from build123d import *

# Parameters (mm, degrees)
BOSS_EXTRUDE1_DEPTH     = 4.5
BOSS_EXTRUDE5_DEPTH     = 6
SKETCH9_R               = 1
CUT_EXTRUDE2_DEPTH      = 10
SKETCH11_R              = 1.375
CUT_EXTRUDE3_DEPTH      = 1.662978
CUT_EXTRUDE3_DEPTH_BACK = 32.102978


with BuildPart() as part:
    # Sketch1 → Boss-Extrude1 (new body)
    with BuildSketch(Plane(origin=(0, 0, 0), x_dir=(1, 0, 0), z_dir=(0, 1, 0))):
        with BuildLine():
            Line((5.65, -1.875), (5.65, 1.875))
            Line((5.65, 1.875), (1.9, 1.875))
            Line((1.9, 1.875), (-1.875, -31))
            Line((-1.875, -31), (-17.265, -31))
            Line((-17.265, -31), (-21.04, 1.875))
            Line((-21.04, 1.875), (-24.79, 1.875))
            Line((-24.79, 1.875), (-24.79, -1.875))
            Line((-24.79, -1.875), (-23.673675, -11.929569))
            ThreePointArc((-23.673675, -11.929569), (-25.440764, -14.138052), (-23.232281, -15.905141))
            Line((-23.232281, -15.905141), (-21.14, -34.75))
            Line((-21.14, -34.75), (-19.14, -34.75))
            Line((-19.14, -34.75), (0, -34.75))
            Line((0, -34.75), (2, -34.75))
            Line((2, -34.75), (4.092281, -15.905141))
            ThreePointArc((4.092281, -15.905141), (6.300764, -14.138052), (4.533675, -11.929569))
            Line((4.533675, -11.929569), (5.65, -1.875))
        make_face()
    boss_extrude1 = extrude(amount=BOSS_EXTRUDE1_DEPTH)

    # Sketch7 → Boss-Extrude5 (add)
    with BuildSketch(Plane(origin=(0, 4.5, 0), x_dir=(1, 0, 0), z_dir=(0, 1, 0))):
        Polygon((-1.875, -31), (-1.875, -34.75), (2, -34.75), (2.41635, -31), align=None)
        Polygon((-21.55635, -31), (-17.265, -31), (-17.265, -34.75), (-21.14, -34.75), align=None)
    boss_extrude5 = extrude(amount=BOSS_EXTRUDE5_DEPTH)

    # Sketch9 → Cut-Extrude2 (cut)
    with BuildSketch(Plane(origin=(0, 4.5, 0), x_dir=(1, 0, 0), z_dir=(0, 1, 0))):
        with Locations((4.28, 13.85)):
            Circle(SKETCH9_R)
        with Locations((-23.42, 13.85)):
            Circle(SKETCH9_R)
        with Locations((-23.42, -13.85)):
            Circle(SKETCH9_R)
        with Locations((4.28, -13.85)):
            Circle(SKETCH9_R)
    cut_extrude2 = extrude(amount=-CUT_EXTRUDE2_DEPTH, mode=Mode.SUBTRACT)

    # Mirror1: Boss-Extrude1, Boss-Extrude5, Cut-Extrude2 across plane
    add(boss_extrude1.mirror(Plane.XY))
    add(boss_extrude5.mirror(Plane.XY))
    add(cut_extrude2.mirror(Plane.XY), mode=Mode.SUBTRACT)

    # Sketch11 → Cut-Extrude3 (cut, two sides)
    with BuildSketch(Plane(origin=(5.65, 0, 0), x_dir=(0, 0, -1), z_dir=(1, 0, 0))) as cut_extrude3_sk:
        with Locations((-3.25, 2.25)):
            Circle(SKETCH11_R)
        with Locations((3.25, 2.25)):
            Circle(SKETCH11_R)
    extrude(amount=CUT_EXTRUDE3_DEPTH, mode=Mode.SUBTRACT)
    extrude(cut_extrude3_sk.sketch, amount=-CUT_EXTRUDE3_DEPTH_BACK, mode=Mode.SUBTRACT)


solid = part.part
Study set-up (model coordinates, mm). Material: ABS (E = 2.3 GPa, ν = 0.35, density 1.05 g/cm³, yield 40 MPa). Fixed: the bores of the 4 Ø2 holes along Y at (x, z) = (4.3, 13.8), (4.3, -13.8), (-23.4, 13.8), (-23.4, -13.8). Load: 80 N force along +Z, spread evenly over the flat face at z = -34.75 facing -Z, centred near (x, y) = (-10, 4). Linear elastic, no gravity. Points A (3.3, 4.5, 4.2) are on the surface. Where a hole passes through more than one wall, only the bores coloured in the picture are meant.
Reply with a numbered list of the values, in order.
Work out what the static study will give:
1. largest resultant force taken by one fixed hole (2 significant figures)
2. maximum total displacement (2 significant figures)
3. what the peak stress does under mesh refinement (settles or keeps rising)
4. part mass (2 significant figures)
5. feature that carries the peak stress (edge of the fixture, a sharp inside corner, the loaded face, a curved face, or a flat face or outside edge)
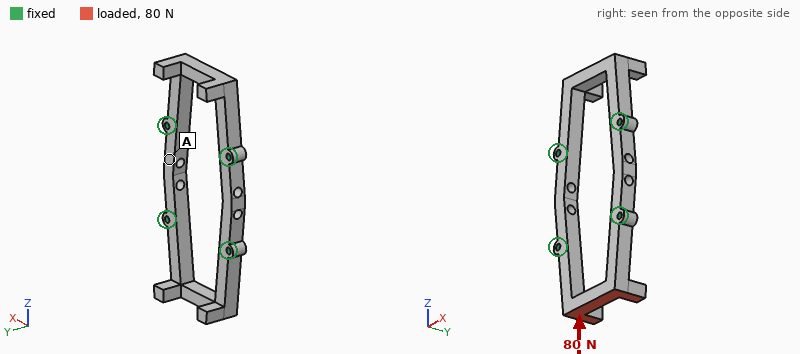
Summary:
1. 40 N
2. 0.27 mm
3. keeps rising
4. 3.7 g
5. edge of the fixture
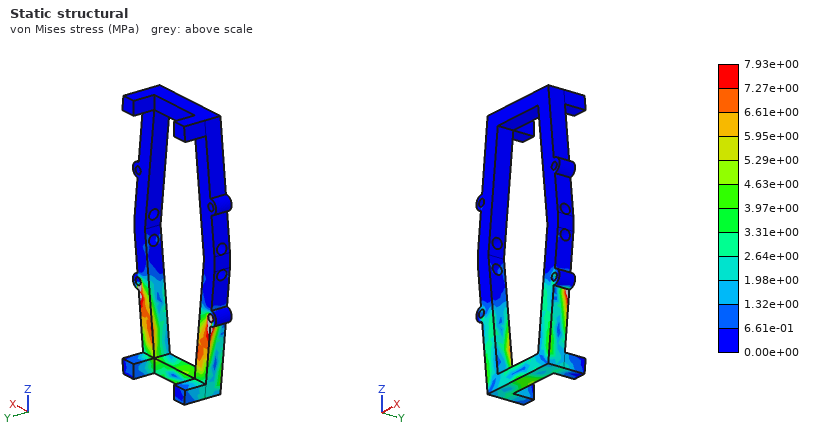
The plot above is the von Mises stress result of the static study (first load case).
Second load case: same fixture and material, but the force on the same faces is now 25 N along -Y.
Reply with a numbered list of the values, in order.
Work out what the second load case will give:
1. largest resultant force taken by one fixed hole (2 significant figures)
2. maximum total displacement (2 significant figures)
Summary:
1. 14 N
2. 0.65 mm
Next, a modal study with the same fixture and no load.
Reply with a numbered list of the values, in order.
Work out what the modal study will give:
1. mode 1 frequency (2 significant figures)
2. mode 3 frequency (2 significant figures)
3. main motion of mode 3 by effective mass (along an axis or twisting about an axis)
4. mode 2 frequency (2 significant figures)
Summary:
1. 1400 Hz
2. 2200 Hz
3. along X
4. 1400 Hz
